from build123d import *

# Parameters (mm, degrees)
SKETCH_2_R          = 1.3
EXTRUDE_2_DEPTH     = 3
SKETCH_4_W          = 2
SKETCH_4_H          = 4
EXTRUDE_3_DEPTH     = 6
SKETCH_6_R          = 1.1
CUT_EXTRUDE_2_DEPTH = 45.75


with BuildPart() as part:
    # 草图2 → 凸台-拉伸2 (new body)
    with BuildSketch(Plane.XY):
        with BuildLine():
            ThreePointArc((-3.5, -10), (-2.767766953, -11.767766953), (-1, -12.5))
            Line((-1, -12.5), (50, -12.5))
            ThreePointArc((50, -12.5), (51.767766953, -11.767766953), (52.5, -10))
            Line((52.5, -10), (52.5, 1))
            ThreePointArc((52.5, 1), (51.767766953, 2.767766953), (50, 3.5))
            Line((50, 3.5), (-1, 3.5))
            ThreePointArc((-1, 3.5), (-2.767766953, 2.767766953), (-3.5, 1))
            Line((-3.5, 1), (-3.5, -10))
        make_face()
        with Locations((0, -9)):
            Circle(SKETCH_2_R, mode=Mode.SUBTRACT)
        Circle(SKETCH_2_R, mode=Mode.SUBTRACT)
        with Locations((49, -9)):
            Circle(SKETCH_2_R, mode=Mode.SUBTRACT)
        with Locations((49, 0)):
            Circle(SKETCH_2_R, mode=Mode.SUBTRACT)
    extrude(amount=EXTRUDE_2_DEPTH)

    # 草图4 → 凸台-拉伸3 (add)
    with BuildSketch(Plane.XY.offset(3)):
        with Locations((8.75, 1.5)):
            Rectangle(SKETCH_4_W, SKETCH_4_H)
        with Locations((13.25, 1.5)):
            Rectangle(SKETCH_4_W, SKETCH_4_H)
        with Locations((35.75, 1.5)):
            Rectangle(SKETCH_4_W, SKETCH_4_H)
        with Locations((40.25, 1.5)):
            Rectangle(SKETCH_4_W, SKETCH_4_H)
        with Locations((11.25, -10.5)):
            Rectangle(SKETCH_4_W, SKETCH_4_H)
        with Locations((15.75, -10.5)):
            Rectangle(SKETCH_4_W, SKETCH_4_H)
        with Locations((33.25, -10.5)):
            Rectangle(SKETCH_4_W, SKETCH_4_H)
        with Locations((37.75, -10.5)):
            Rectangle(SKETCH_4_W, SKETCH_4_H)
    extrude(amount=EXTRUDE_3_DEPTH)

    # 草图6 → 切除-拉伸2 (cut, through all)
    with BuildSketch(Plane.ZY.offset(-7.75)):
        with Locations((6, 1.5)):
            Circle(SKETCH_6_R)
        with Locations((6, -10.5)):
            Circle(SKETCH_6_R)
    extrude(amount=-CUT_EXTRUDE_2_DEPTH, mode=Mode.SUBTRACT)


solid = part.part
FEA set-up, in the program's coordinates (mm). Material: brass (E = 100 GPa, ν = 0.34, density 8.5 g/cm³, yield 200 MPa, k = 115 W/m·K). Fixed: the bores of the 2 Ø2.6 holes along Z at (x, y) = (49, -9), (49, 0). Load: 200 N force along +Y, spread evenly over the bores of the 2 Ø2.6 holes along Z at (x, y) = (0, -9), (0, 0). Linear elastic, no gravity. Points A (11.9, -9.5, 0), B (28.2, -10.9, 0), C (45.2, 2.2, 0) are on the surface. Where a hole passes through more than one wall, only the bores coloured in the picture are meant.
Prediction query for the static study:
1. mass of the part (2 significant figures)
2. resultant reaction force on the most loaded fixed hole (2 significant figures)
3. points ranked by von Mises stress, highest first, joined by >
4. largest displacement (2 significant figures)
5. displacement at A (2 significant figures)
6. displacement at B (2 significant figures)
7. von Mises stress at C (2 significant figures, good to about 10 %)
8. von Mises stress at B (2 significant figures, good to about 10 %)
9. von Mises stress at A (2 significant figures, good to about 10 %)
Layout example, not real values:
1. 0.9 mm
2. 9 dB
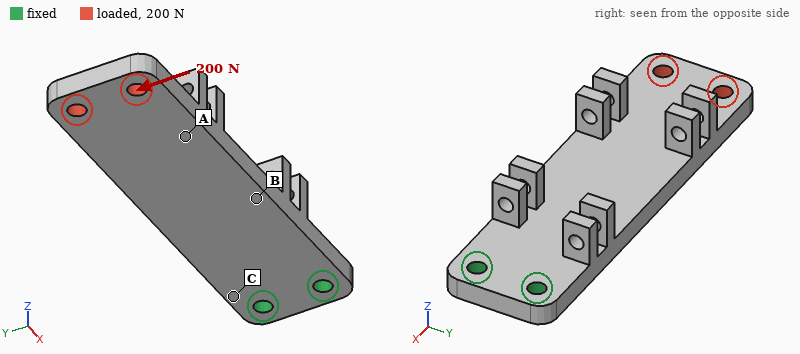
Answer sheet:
1. 25 g
2. 940 N
3. C > B > A
4. 94 µm
5. 57 µm
6. 24 µm
7. 54 MPa
8. 35 MPa
9. 14 MPa
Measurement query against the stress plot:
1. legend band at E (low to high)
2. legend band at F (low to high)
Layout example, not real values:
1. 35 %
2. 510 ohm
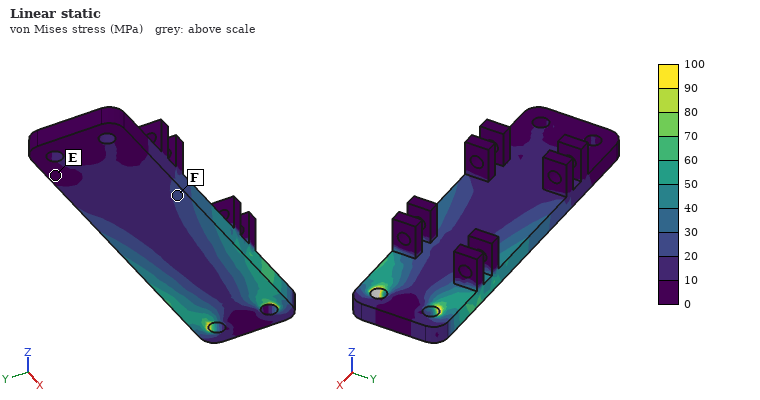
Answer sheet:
1. 0 to 10 MPa
2. 20 to 30 MPa
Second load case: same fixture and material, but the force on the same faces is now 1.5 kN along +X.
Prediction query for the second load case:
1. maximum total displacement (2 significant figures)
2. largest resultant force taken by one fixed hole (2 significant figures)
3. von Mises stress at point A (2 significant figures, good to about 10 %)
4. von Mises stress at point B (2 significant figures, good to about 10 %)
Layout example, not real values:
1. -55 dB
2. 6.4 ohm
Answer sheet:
1. 18 µm
2. 760 N
3. 33 MPa
4. 31 MPa
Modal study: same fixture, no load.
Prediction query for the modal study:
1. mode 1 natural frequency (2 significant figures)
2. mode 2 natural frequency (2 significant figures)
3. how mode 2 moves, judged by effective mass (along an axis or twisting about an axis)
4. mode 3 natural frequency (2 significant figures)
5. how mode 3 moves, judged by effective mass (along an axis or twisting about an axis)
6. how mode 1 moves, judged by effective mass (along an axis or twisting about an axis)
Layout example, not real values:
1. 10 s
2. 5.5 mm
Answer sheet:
1. 610 Hz
2. 2900 Hz
3. along Y
4. 3400 Hz
5. twisting about X
6. along Z
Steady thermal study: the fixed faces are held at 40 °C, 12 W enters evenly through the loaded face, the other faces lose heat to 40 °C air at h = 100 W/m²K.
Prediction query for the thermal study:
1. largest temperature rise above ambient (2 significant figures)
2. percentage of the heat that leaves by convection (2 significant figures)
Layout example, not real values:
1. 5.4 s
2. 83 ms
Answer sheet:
1. 63 K
2. 59 %
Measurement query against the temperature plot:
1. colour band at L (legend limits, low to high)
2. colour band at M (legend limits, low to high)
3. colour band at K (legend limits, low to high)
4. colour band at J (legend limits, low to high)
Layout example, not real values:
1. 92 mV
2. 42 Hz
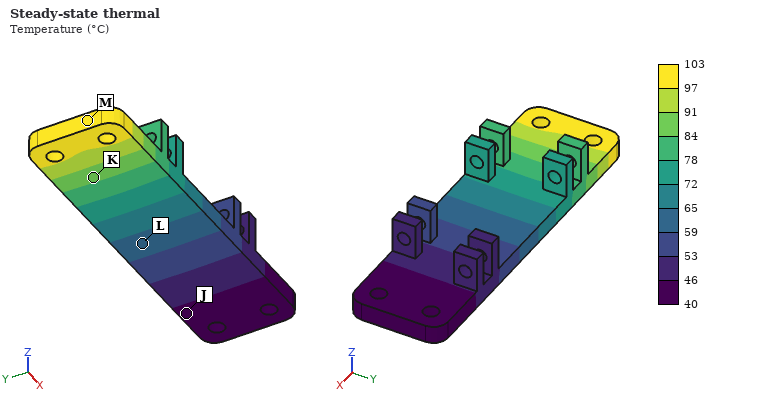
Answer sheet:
1. 59 to 65 °C
2. 97 to 103 °C
3. 84 to 91 °C
4. 40 to 46 °C
